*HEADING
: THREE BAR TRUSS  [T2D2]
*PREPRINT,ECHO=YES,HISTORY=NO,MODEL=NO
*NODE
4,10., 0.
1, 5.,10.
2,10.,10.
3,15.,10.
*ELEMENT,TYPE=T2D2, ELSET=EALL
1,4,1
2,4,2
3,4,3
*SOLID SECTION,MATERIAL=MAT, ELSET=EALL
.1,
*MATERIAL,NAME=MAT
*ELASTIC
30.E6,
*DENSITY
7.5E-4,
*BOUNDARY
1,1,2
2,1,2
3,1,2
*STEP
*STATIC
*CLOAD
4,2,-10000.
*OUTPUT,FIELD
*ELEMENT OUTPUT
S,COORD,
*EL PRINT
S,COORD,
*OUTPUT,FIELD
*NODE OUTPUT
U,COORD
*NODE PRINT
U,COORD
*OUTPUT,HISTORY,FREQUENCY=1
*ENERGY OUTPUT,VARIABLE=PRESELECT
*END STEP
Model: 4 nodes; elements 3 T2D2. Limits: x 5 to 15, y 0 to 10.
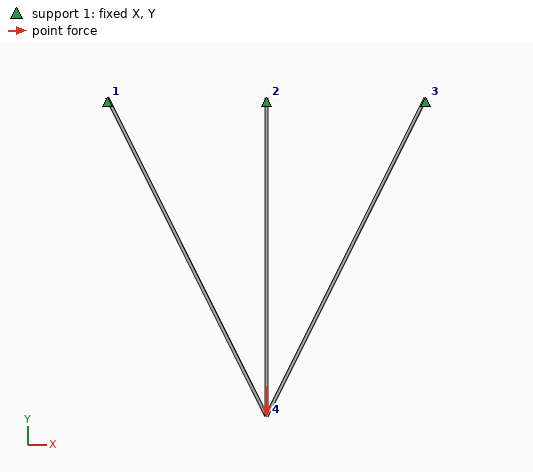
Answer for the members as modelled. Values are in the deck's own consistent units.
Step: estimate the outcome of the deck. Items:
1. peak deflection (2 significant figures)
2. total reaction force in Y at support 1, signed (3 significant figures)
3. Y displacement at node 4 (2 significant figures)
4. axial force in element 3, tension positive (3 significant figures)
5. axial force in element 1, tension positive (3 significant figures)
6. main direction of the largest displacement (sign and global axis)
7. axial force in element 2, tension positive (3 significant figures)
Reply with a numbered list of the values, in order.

1. 0.014
2. 10000
3. -0.014
4. 3290
5. 3290
6. -Y
7. 4110
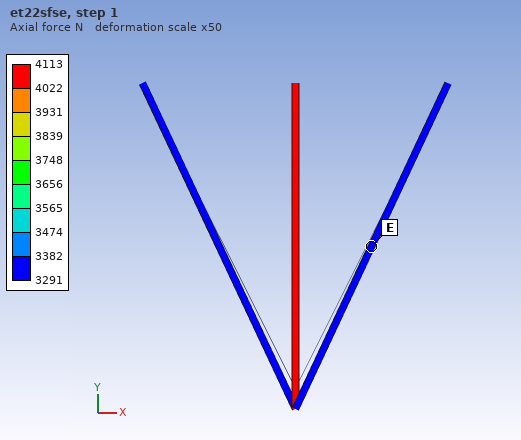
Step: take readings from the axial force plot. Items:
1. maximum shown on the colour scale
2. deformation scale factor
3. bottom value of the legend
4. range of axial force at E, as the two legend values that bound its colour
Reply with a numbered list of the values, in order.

1. 4113
2. 50
3. 3291
4. 3291 to 3382
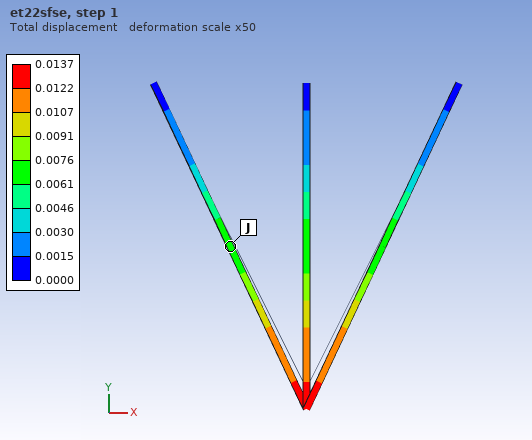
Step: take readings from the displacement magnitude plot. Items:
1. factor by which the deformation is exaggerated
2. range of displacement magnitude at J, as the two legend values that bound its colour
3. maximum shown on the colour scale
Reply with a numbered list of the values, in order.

1. 50
2. 0.0061 to 0.0076
3. 0.0137
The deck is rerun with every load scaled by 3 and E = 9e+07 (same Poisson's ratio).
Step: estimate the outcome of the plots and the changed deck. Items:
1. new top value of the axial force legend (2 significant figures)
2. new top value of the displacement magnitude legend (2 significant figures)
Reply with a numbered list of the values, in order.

1. 12000
2. 0.014
